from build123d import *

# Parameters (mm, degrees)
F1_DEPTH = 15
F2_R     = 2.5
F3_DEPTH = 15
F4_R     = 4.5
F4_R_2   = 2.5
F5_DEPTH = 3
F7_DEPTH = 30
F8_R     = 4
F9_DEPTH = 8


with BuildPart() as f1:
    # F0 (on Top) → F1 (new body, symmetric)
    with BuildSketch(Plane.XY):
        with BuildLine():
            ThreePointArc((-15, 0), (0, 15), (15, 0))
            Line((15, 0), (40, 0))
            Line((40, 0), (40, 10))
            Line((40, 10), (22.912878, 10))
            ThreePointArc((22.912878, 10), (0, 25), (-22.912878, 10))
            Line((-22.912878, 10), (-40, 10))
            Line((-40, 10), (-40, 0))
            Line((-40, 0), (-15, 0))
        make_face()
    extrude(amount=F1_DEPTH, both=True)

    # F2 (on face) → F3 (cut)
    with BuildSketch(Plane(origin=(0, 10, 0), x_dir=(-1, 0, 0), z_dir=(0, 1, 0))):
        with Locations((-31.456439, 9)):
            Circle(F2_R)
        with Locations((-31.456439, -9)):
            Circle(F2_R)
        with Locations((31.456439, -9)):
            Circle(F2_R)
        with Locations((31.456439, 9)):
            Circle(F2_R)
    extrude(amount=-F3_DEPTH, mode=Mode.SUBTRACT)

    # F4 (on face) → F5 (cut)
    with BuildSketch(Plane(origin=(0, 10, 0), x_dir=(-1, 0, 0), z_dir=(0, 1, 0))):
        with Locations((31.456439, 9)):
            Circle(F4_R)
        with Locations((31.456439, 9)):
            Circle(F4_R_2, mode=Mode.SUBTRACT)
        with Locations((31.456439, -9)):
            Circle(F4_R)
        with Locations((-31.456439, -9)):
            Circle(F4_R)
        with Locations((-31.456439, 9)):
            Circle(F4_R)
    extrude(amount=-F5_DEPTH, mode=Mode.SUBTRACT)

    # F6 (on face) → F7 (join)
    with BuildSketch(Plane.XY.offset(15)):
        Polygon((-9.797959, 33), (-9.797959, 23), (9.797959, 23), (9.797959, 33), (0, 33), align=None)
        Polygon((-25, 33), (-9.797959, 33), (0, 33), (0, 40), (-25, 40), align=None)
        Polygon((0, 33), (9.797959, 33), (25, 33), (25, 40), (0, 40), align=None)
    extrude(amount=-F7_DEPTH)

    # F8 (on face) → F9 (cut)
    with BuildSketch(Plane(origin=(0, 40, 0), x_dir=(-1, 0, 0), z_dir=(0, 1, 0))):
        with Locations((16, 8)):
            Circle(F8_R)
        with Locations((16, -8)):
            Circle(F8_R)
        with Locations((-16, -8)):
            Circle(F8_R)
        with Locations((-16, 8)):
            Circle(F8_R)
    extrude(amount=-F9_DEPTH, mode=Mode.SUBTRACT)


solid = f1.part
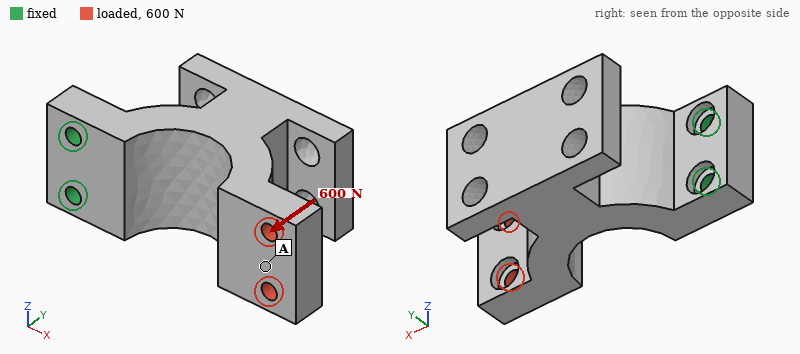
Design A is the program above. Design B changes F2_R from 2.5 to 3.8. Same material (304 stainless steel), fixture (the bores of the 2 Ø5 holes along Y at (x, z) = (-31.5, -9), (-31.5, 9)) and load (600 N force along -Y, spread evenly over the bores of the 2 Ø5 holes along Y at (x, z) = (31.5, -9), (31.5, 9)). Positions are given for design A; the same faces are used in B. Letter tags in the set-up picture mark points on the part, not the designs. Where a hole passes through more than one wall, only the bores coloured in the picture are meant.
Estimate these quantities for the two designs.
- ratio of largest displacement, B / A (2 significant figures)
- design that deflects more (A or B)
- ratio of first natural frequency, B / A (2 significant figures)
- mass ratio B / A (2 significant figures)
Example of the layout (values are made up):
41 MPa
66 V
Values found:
0.87
A
1.1
0.98
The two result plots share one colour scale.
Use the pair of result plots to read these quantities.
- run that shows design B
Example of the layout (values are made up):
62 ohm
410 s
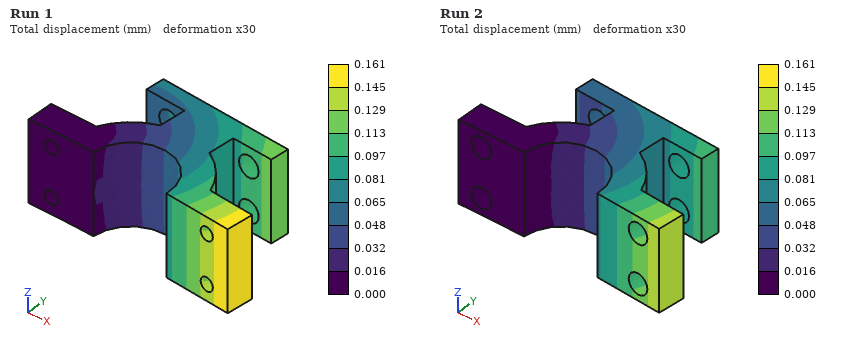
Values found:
Run 2
